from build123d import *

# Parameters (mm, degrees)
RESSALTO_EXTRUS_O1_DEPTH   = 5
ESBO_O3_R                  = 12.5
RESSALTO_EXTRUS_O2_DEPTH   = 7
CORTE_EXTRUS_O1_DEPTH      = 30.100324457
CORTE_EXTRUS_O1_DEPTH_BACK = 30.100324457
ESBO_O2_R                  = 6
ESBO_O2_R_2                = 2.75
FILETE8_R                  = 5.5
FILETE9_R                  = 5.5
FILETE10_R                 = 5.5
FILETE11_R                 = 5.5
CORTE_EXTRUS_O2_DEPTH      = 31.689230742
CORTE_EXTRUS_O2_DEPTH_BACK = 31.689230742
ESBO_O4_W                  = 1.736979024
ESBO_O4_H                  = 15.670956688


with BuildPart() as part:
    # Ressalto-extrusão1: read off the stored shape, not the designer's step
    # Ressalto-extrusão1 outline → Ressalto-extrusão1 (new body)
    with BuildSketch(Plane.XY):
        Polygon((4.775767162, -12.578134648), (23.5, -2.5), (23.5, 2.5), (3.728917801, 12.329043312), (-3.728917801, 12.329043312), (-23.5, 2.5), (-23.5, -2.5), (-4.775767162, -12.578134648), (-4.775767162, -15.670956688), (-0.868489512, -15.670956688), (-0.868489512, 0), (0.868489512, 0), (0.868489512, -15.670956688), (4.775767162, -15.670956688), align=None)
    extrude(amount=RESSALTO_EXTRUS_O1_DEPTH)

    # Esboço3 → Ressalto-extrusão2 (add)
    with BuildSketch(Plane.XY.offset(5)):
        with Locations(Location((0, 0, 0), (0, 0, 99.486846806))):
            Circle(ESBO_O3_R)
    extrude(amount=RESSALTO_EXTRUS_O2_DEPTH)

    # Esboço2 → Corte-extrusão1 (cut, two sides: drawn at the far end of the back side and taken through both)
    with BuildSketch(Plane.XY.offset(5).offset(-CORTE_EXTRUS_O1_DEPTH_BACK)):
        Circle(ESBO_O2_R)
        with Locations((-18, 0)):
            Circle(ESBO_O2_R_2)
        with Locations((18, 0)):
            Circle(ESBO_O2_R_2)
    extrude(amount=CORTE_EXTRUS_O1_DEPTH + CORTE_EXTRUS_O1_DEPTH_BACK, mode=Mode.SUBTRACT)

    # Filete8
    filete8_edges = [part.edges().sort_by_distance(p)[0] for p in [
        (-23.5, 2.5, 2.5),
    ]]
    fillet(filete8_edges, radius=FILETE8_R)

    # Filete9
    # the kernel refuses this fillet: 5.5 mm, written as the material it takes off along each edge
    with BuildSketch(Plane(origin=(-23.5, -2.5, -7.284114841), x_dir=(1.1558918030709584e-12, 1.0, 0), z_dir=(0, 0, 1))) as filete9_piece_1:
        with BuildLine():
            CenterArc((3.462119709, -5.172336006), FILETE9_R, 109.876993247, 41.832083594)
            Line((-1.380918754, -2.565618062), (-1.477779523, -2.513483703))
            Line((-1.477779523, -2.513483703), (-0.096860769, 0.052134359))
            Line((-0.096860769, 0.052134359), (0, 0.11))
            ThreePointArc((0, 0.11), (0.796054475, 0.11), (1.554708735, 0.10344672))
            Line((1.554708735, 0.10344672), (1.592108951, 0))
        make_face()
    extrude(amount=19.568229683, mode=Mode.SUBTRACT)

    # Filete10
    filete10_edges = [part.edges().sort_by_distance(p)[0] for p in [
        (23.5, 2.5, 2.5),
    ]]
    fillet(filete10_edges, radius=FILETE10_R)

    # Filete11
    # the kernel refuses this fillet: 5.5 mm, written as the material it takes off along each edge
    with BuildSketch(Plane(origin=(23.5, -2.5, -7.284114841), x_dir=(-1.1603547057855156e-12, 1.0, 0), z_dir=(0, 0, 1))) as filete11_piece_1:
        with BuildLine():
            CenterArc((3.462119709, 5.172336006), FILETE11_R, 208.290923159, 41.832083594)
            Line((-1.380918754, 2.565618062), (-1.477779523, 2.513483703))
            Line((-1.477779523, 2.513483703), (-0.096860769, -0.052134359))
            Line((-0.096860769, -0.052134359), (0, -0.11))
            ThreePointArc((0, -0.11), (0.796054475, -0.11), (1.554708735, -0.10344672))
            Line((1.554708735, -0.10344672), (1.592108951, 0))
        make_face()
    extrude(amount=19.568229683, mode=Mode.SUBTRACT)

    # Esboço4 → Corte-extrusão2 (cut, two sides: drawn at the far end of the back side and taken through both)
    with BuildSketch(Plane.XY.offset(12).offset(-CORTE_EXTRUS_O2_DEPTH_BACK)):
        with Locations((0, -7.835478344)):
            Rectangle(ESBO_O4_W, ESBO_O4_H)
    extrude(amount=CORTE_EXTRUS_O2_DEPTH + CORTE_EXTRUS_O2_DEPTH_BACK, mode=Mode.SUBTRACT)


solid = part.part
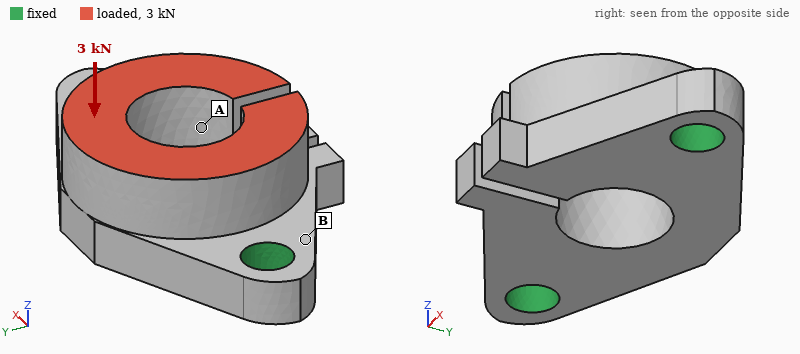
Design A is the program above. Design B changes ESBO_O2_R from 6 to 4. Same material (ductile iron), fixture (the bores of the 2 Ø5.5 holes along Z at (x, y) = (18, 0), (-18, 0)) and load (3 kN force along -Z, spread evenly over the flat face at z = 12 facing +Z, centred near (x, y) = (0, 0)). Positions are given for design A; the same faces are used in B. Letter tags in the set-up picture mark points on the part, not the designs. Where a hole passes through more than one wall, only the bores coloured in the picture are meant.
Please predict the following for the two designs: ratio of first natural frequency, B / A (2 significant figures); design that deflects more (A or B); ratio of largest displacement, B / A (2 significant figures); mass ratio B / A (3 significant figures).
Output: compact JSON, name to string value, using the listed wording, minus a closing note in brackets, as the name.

{"ratio of first natural frequency, B / A": "0.99", "design that deflects more": "A", "ratio of largest displacement, B / A": "0.70", "mass ratio B / A": "1.12"}
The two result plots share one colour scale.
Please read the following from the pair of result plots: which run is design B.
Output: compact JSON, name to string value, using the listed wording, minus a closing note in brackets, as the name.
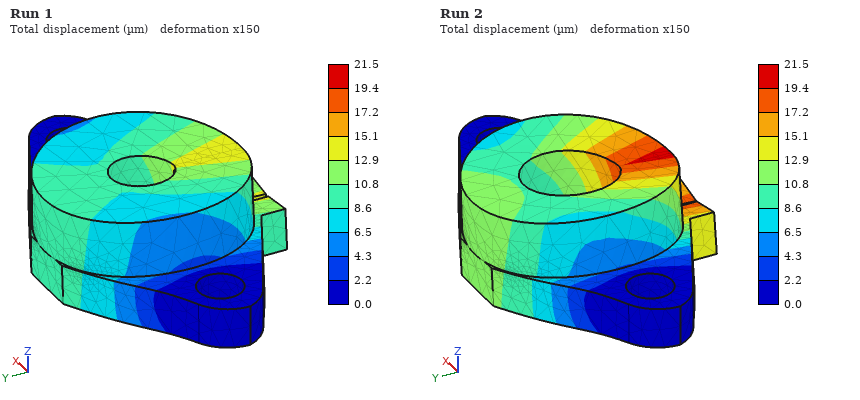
{"which run is design B": "Run 1"}
